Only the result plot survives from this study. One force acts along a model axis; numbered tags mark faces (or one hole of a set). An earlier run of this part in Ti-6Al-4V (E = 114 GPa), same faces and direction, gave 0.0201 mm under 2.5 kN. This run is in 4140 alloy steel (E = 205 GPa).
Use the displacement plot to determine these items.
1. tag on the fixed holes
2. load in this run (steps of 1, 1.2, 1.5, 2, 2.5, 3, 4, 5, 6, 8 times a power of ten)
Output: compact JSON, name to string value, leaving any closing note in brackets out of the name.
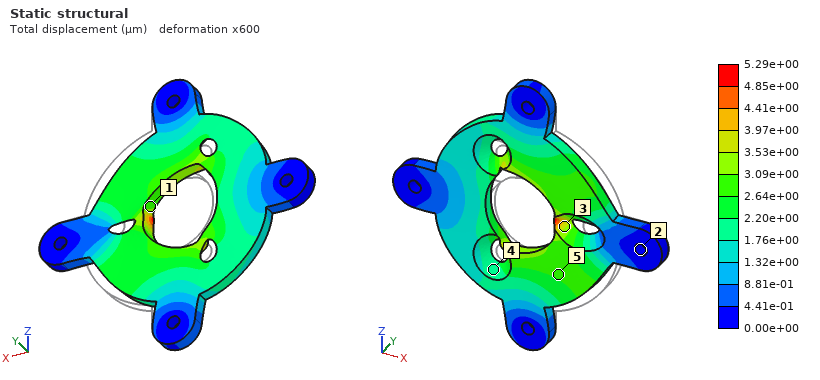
{"tag on the fixed holes": "2", "load in this run": "1.2 kN"}
